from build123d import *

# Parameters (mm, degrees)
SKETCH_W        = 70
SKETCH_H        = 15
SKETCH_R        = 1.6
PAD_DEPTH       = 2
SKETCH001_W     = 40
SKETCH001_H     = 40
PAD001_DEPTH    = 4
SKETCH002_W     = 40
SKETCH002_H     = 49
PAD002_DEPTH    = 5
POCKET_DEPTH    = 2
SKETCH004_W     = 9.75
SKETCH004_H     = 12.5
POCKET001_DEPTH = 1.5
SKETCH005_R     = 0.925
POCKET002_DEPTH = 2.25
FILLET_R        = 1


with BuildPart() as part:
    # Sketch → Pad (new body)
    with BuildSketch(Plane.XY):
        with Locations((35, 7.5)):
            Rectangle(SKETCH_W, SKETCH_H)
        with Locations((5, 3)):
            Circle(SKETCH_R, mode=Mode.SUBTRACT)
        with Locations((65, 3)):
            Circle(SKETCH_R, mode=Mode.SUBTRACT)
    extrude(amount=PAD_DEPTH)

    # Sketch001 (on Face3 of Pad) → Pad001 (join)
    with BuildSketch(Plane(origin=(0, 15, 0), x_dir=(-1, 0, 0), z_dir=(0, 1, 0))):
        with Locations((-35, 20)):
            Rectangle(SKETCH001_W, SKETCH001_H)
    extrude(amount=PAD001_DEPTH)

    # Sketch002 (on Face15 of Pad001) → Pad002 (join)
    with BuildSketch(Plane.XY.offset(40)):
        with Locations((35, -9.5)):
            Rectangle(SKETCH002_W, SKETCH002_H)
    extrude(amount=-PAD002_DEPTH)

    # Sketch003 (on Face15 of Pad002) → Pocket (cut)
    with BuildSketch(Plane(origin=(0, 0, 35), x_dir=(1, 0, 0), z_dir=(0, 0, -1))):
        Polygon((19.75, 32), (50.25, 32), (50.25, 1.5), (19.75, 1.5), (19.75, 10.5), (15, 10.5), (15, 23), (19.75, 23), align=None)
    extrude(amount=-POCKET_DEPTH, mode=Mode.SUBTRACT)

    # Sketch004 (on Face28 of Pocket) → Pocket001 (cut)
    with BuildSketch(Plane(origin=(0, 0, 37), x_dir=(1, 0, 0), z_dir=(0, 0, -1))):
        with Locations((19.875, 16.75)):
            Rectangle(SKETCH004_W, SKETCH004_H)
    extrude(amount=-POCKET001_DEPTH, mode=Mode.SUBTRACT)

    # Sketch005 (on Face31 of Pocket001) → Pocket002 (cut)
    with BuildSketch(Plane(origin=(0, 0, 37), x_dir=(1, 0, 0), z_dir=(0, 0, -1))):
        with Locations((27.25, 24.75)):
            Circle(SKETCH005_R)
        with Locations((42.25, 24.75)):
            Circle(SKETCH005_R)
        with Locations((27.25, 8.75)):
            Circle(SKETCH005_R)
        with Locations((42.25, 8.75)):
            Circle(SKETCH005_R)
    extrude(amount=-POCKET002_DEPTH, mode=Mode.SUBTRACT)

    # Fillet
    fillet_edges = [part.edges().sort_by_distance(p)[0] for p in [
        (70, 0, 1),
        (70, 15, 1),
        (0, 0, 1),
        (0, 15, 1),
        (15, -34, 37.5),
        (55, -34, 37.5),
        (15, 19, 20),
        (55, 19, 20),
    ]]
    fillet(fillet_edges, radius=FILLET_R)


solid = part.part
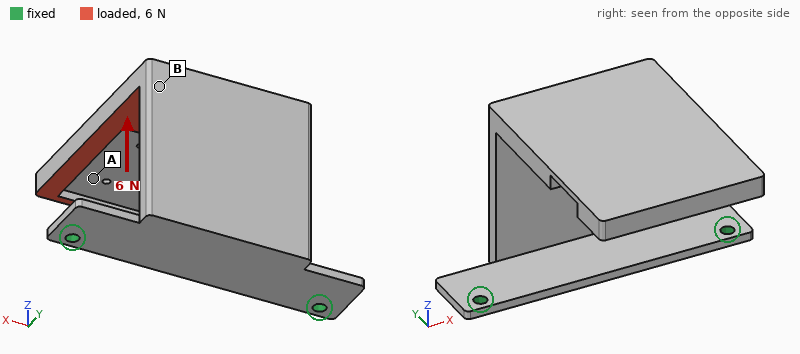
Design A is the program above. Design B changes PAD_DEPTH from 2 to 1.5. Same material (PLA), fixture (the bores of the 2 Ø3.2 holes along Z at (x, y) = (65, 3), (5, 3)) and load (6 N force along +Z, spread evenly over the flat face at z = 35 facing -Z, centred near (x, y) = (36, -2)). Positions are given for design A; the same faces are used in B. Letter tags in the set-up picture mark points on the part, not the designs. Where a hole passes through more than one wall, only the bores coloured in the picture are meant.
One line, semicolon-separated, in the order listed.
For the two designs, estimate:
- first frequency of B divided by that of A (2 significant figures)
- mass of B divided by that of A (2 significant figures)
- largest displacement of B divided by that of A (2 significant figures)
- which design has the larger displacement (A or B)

0.68; 0.97; 1.9; B
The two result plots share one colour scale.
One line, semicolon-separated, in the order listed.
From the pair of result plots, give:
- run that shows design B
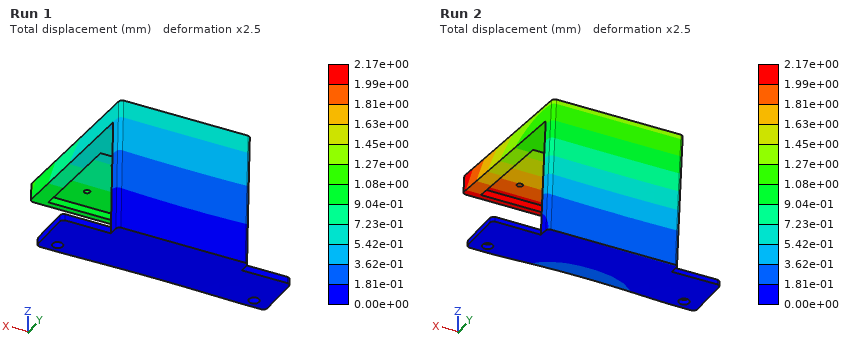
Run 2
